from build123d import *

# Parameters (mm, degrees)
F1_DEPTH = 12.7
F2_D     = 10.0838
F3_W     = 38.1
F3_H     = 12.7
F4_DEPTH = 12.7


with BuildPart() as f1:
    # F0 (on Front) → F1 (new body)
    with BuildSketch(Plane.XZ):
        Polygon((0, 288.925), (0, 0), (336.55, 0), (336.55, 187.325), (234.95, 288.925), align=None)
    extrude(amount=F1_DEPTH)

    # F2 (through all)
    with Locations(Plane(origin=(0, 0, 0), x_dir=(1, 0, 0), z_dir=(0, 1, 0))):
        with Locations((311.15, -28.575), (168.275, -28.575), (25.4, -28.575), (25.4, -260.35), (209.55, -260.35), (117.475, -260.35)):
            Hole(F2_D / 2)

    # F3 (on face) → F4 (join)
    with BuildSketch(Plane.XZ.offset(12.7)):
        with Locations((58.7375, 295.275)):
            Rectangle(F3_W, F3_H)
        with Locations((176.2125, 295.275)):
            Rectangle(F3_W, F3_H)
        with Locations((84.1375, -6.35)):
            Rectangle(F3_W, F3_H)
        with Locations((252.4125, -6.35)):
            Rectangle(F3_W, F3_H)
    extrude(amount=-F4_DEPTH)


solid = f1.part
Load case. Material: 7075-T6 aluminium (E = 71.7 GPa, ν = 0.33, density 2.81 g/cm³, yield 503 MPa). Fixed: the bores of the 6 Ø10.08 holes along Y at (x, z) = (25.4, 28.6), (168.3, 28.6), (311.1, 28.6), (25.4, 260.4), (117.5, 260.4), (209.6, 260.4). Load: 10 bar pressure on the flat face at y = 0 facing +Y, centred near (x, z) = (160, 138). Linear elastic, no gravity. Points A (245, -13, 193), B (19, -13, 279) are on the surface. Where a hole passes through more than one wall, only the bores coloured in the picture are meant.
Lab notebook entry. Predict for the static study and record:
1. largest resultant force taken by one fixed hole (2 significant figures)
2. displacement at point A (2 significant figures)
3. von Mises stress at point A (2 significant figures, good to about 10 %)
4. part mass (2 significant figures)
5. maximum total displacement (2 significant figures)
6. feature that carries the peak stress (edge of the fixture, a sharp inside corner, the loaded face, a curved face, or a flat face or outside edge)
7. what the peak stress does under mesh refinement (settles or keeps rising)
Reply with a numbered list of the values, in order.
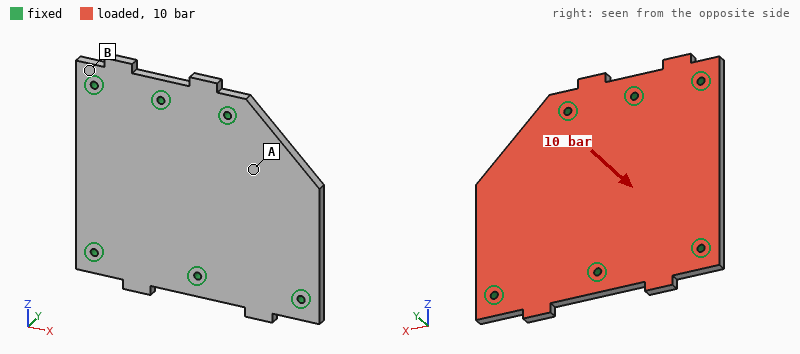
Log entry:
1. 21 kN
2. 0.93 mm
3. 91 MPa
4. 3.3 kg
5. 1.9 mm
6. edge of the fixture
7. keeps rising
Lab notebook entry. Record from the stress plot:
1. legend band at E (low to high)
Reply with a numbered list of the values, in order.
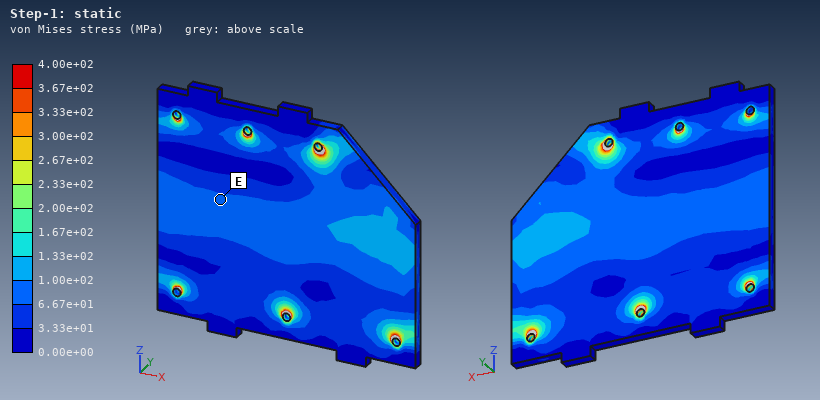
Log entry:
1. 6.67e+01 to 1.00e+02 MPa
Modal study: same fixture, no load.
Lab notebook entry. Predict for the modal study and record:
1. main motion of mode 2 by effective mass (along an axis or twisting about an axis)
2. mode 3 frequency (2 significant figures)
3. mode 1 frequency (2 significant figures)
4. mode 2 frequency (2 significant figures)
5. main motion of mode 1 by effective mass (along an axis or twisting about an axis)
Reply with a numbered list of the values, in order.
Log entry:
1. along Y
2. 1500 Hz
3. 820 Hz
4. 1100 Hz
5. along Y
